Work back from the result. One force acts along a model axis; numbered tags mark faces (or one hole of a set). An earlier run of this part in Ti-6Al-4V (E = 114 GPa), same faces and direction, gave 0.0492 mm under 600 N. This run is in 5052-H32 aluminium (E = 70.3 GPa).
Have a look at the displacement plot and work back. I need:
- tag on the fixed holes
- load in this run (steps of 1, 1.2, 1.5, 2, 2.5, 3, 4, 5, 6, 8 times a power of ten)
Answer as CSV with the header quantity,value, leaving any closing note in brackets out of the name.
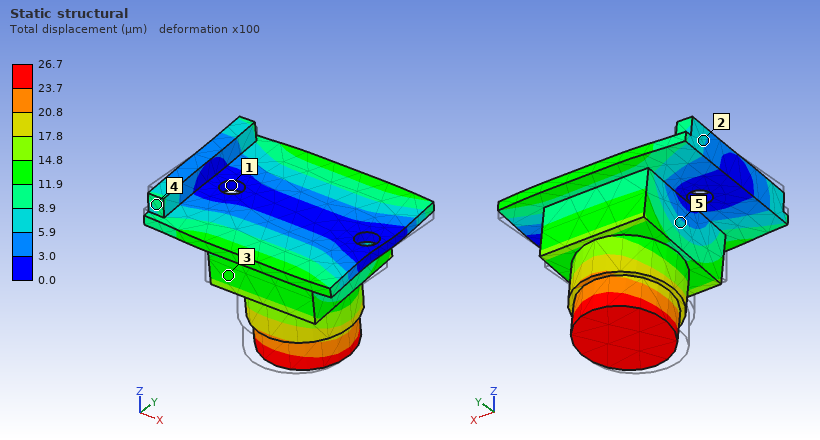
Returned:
quantity,value
tag on the fixed holes,1
load in this run,200 N
